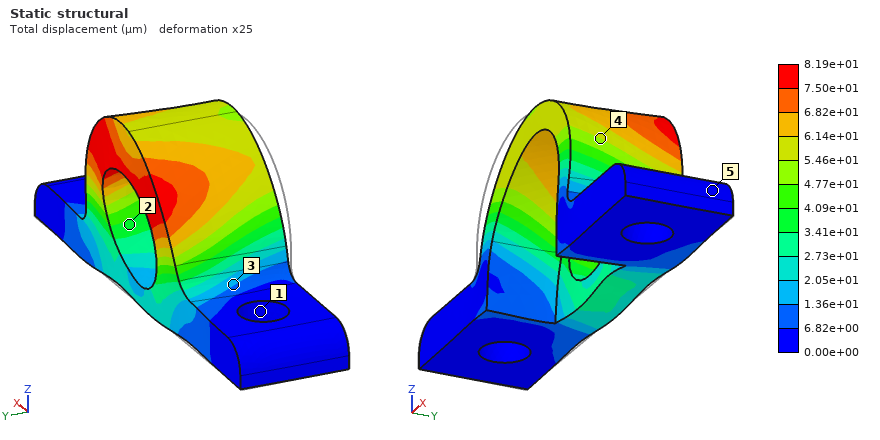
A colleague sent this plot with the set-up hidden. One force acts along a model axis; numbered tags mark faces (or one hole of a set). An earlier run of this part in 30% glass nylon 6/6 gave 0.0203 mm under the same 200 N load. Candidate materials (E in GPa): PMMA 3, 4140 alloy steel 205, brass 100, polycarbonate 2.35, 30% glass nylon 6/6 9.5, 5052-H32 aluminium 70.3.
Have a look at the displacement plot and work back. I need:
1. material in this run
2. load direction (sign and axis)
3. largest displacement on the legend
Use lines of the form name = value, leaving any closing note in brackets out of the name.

material in this run = polycarbonate
load direction = +X
largest displacement on the legend = 8.19e+01 µm
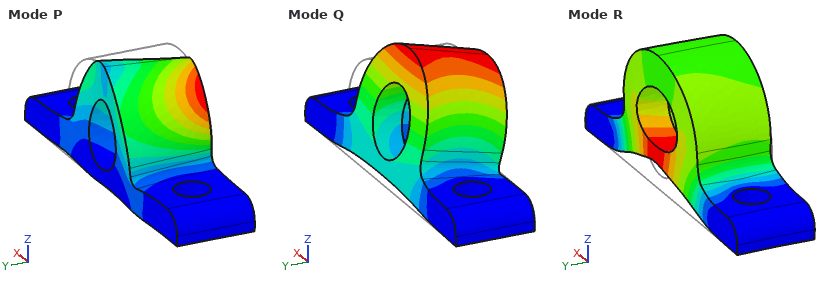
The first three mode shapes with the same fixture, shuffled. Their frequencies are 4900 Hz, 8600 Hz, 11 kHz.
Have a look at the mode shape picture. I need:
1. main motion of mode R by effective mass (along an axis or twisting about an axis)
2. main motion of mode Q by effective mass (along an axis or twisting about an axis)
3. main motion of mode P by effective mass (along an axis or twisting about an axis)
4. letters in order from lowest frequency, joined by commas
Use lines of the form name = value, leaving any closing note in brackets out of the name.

main motion of mode R by effective mass = along Z
main motion of mode Q by effective mass = along Y
main motion of mode P by effective mass = along X
letters in order from lowest frequency, joined by commas = Q, P, R
